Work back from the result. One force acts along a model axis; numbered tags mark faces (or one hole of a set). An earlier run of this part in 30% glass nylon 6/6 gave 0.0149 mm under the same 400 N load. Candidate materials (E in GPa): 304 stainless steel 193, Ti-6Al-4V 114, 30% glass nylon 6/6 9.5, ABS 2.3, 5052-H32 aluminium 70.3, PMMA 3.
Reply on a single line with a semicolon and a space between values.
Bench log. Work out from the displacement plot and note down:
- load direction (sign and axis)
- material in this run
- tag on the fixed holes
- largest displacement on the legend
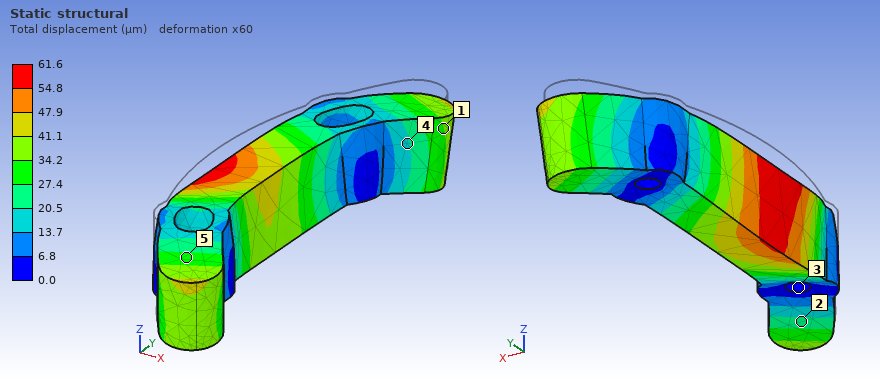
-Z; ABS; 3; 61.6 µm
